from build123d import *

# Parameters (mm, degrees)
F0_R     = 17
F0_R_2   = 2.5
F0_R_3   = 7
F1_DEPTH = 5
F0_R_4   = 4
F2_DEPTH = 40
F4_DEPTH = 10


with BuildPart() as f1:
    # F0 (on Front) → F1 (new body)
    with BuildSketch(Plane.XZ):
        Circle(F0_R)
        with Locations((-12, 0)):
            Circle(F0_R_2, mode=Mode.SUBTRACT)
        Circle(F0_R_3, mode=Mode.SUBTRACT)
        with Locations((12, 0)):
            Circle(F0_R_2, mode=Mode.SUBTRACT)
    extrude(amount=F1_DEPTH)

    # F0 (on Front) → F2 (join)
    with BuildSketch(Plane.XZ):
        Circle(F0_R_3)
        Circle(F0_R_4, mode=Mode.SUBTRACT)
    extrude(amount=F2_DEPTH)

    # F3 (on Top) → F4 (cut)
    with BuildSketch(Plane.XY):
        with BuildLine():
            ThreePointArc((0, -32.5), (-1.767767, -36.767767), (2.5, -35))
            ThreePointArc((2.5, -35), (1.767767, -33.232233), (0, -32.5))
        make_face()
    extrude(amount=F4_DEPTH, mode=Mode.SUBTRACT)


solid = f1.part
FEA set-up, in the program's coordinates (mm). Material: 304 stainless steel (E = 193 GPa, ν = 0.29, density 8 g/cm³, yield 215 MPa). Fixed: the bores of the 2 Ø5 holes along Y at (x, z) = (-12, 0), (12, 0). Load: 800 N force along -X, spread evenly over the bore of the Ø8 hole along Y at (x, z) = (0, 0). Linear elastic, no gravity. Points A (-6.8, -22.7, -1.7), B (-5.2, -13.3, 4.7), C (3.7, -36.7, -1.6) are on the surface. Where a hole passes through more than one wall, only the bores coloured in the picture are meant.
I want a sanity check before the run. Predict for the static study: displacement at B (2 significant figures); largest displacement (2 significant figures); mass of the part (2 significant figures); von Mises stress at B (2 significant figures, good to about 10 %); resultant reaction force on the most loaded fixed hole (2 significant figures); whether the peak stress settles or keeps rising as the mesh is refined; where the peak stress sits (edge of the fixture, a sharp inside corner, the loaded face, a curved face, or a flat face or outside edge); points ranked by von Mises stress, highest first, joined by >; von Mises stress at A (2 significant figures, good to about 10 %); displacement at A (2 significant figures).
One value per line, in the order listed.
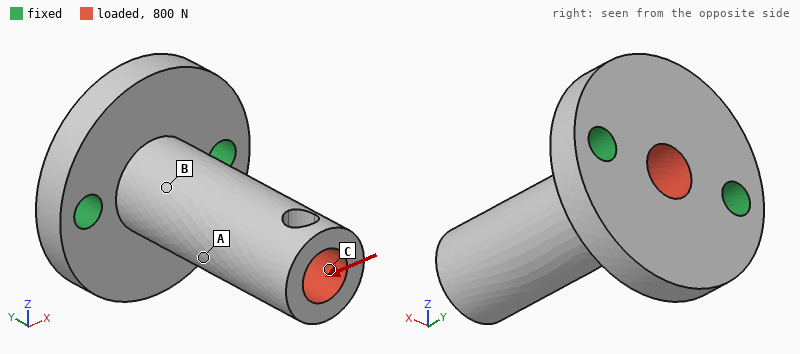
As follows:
5.0 µm
22 µm
61 g
22 MPa
870 N
keeps rising
edge of the fixture
B > A > C
12 MPa
11 µm
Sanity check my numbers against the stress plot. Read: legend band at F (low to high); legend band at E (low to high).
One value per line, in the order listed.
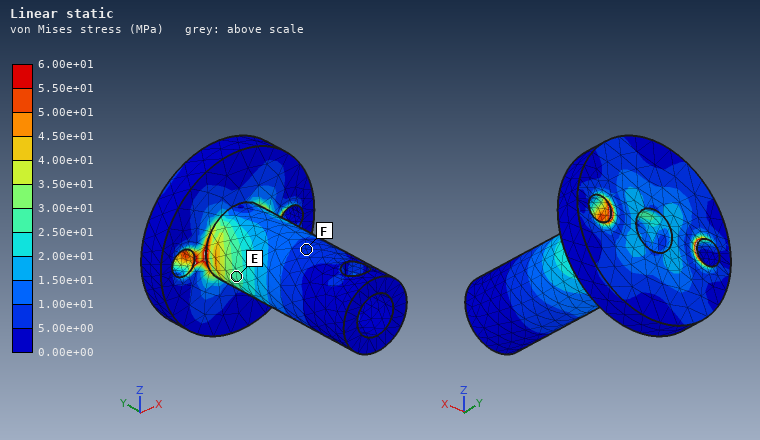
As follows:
5.00e+00 to 1.00e+01 MPa
2.50e+01 to 3.00e+01 MPa
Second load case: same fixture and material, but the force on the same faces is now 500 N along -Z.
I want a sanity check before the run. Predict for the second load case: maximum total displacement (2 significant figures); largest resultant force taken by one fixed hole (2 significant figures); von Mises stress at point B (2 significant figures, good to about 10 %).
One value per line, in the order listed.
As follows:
27 µm
250 N
13 MPa
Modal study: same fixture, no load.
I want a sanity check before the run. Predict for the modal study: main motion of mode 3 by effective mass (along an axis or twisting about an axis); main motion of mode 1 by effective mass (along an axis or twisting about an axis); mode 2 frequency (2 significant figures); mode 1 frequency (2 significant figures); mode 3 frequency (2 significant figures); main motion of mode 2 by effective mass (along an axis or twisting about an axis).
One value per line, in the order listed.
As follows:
along Y
along Z
6400 Hz
4500 Hz
17 kHz
along X
